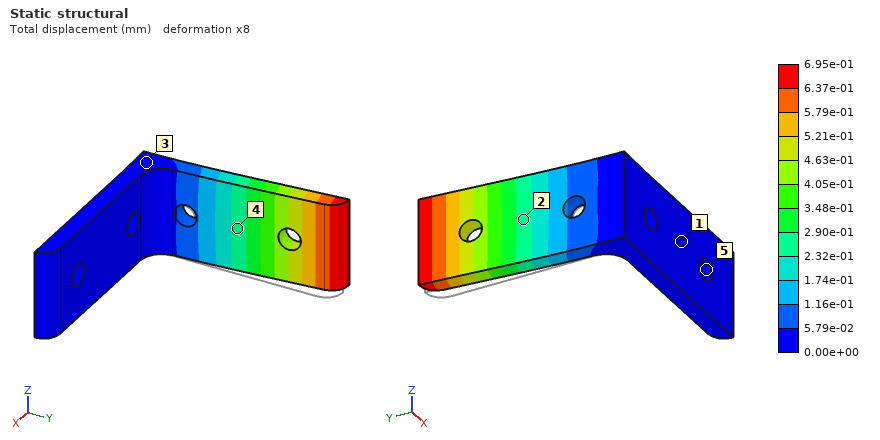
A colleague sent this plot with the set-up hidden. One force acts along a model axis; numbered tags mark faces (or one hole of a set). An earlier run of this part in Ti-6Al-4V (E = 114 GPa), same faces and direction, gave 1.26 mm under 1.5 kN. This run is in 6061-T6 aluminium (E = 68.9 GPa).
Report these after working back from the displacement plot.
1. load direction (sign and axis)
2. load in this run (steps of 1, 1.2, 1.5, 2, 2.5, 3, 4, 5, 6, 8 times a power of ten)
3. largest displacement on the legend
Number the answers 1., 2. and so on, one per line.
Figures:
1. -X
2. 500 N
3. 6.95e-01 mm
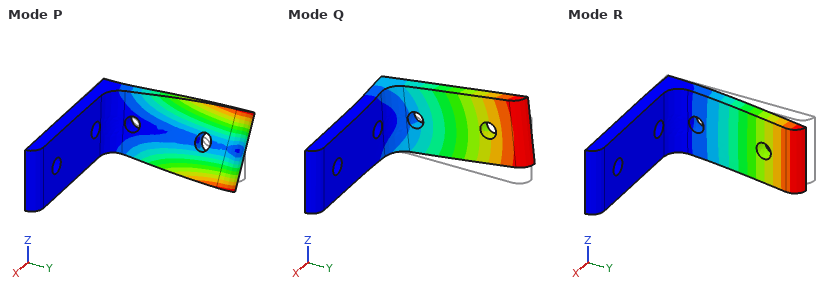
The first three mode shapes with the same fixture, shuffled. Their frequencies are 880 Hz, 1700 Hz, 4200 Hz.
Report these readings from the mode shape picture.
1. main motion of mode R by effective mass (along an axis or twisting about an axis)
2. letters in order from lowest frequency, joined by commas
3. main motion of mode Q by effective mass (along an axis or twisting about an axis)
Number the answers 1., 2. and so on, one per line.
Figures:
1. along X
2. R, Q, P
3. along Z
